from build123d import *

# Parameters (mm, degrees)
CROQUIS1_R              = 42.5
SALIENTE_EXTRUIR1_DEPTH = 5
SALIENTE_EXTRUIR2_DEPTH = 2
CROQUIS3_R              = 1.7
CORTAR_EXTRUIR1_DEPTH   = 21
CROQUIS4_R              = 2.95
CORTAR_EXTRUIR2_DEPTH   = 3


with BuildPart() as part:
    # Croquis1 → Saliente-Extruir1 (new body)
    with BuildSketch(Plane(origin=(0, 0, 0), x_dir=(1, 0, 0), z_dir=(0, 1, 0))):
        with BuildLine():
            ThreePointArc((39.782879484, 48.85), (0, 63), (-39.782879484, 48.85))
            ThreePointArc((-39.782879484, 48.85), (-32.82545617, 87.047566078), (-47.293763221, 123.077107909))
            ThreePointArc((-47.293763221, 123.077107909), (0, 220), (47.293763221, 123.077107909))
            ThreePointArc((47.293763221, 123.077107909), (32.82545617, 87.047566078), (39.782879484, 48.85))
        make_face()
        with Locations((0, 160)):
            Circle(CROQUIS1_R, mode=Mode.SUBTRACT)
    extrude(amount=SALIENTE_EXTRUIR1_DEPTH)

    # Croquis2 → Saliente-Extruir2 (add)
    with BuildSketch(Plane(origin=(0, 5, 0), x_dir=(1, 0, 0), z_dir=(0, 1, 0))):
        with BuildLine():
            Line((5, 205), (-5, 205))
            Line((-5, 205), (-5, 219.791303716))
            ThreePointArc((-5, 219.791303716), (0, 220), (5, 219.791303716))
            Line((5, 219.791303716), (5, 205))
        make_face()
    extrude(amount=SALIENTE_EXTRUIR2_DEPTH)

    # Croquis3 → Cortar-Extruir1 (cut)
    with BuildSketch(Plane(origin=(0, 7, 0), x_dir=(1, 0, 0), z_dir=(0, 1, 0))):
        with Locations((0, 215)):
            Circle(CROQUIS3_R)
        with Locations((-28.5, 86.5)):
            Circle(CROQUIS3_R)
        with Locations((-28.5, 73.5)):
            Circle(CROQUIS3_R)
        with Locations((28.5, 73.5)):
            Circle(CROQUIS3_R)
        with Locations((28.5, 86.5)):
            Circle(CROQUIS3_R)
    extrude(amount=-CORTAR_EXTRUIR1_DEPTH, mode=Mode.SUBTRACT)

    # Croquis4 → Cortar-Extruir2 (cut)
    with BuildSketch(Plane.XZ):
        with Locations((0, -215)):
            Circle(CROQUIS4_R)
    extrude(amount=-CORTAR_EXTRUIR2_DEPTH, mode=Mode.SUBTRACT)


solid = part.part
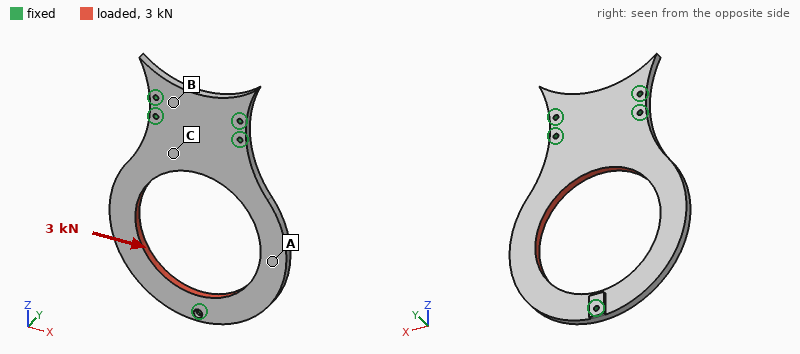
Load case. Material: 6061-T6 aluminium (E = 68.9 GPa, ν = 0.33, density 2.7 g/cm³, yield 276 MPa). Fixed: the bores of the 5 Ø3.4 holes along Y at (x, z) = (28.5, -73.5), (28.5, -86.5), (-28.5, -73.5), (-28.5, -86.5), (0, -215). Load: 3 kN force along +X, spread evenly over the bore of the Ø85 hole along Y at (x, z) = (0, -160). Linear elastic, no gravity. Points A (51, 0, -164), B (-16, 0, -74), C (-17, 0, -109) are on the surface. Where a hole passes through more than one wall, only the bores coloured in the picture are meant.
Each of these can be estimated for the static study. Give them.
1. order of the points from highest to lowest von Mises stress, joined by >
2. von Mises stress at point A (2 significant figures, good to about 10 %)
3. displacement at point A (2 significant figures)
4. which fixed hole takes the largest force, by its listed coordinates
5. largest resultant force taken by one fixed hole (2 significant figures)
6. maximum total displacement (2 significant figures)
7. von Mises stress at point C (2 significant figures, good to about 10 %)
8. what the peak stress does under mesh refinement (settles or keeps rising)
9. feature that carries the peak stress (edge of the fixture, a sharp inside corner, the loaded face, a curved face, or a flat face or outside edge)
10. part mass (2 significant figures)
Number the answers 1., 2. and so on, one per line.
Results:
1. C > A > B
2. 5.3 MPa
3. 34 µm
4. (0, -215)
5. 1.5 kN
6. 43 µm
7. 9.5 MPa
8. keeps rising
9. edge of the fixture
10. 120 g
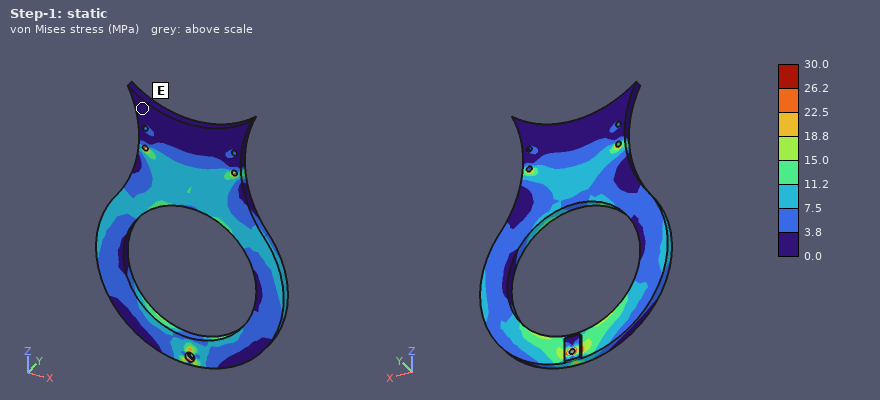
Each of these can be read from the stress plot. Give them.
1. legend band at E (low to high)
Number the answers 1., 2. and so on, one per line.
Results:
1. 0.0 to 3.8 MPa
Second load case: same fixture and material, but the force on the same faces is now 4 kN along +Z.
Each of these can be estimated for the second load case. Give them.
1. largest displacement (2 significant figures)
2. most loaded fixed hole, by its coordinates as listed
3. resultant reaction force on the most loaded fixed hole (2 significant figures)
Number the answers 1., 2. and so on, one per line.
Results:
1. 27 µm
2. (0, -215)
3. 1.4 kN
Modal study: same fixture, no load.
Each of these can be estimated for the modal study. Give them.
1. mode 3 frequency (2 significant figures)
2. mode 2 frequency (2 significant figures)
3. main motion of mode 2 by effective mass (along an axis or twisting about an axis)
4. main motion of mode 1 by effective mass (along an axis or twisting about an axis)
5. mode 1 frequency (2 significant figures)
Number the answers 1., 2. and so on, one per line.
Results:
1. 2500 Hz
2. 960 Hz
3. along Y
4. twisting about Z
5. 880 Hz
